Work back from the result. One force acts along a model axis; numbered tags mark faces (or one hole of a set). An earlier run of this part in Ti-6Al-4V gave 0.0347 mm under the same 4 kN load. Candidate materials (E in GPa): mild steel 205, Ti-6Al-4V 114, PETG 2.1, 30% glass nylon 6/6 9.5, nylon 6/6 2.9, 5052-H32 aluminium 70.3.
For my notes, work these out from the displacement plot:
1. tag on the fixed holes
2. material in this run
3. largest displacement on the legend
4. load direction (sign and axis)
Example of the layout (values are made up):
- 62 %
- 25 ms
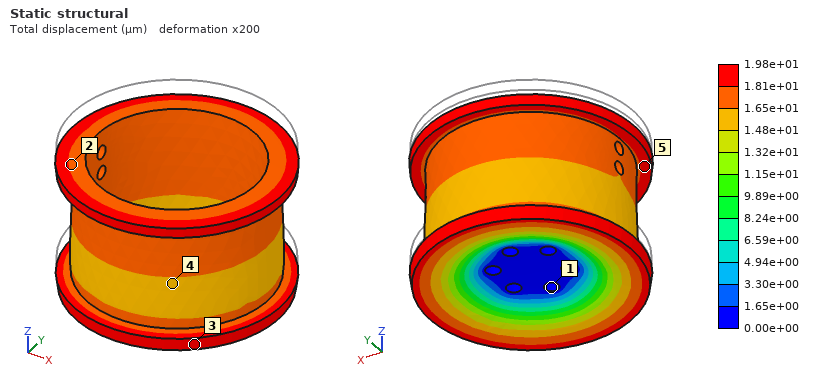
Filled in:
- 1
- mild steel
- 1.98e+01 µm
- -Z
